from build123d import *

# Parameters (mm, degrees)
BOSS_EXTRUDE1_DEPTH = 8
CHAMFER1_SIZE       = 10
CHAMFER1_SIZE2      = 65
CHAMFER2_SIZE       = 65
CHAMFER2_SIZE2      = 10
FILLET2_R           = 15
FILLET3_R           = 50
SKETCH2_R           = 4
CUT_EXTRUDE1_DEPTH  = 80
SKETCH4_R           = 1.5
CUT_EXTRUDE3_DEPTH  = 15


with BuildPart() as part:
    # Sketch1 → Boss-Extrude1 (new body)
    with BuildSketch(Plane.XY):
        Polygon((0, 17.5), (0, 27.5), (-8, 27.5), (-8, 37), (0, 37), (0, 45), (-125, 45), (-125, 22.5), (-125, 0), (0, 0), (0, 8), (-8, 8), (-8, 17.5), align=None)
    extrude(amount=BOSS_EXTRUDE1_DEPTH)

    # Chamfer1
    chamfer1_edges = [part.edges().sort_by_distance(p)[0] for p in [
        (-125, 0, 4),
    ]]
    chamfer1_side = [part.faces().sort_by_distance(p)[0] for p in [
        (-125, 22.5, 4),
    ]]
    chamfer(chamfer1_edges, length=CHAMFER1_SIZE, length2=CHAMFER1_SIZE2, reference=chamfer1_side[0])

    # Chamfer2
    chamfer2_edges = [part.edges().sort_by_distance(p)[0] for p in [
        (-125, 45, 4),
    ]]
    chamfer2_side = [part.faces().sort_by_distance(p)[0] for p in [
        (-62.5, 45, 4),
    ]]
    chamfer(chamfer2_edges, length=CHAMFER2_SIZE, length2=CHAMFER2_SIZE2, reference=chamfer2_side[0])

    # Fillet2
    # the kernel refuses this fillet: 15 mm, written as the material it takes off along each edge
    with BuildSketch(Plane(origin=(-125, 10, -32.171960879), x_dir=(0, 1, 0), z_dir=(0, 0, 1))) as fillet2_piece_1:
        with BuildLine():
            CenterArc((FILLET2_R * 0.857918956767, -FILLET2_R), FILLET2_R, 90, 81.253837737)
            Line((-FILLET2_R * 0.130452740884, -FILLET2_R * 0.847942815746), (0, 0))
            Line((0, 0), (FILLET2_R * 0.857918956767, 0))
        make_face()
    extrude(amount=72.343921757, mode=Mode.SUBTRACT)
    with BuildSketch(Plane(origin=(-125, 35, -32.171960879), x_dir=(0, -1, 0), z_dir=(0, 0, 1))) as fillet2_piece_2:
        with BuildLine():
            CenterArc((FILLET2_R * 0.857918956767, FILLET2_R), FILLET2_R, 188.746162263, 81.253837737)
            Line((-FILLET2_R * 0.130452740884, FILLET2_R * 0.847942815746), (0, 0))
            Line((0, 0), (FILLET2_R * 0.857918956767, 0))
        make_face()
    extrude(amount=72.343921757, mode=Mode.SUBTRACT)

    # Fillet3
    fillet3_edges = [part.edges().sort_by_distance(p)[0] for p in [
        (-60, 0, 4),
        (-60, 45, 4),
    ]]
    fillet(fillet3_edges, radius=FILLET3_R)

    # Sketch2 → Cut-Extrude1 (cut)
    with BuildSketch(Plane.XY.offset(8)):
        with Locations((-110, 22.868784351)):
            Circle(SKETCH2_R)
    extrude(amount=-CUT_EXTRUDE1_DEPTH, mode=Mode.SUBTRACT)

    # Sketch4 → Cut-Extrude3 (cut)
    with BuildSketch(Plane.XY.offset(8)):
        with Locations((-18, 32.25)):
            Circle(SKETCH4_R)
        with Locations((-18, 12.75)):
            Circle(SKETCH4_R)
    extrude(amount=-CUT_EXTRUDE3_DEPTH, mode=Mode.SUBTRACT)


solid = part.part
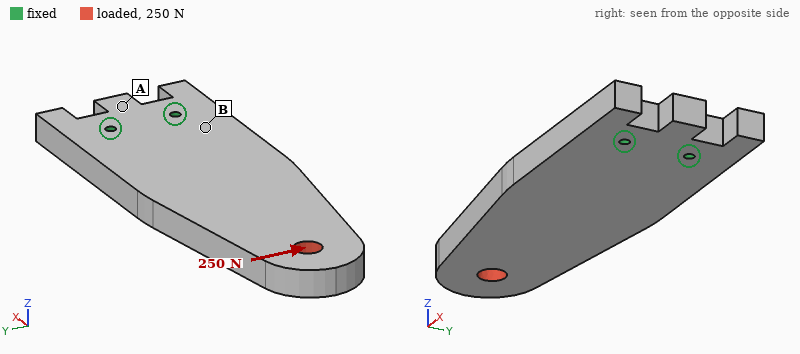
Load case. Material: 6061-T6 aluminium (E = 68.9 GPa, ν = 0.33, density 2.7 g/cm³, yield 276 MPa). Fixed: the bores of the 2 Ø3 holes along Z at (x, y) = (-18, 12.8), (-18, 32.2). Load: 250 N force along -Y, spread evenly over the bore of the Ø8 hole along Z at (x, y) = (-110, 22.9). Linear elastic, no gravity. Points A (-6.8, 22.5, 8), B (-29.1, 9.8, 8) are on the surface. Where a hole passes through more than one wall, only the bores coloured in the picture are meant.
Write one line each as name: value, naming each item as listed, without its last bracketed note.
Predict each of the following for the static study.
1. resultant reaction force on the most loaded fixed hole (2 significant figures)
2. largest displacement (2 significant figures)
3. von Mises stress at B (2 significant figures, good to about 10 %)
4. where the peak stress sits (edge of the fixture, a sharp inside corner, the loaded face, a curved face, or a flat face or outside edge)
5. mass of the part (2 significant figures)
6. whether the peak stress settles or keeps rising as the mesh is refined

resultant reaction force on the most loaded fixed hole: 1.1 kN
largest displacement: 36 µm
von Mises stress at B: 6.1 MPa
where the peak stress sits: edge of the fixture
mass of the part: 100 g
whether the peak stress settles or keeps rising as the mesh is refined: keeps rising
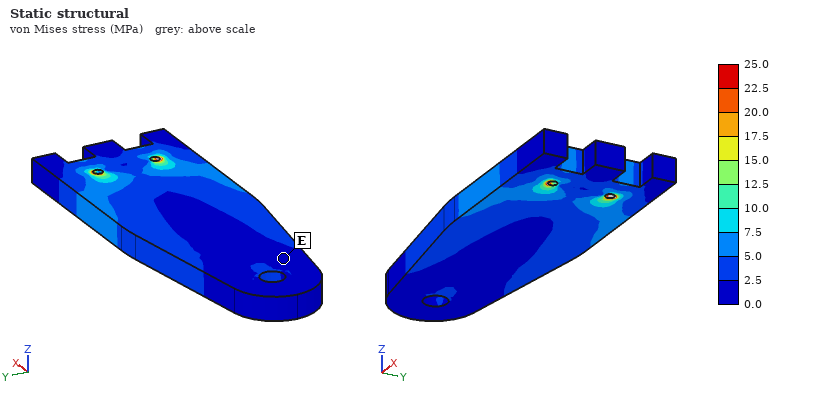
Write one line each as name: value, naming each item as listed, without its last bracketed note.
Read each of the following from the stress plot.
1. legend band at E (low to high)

legend band at E: 0.0 to 2.5 MPa
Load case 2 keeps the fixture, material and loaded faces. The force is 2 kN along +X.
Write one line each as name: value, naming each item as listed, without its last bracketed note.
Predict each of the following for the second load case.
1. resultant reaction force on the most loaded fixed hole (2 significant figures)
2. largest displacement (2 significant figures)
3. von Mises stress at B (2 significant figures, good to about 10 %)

resultant reaction force on the most loaded fixed hole: 1.0 kN
largest displacement: 11 µm
von Mises stress at B: 6.5 MPa
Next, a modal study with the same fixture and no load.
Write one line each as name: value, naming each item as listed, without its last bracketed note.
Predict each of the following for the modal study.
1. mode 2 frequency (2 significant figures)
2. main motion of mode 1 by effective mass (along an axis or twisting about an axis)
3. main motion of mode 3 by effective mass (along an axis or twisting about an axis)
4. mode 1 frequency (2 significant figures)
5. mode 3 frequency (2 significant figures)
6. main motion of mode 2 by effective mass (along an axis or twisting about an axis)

mode 2 frequency: 2700 Hz
main motion of mode 1 by effective mass: along Z
main motion of mode 3 by effective mass: twisting about X
mode 1 frequency: 680 Hz
mode 3 frequency: 3600 Hz
main motion of mode 2 by effective mass: along Y
